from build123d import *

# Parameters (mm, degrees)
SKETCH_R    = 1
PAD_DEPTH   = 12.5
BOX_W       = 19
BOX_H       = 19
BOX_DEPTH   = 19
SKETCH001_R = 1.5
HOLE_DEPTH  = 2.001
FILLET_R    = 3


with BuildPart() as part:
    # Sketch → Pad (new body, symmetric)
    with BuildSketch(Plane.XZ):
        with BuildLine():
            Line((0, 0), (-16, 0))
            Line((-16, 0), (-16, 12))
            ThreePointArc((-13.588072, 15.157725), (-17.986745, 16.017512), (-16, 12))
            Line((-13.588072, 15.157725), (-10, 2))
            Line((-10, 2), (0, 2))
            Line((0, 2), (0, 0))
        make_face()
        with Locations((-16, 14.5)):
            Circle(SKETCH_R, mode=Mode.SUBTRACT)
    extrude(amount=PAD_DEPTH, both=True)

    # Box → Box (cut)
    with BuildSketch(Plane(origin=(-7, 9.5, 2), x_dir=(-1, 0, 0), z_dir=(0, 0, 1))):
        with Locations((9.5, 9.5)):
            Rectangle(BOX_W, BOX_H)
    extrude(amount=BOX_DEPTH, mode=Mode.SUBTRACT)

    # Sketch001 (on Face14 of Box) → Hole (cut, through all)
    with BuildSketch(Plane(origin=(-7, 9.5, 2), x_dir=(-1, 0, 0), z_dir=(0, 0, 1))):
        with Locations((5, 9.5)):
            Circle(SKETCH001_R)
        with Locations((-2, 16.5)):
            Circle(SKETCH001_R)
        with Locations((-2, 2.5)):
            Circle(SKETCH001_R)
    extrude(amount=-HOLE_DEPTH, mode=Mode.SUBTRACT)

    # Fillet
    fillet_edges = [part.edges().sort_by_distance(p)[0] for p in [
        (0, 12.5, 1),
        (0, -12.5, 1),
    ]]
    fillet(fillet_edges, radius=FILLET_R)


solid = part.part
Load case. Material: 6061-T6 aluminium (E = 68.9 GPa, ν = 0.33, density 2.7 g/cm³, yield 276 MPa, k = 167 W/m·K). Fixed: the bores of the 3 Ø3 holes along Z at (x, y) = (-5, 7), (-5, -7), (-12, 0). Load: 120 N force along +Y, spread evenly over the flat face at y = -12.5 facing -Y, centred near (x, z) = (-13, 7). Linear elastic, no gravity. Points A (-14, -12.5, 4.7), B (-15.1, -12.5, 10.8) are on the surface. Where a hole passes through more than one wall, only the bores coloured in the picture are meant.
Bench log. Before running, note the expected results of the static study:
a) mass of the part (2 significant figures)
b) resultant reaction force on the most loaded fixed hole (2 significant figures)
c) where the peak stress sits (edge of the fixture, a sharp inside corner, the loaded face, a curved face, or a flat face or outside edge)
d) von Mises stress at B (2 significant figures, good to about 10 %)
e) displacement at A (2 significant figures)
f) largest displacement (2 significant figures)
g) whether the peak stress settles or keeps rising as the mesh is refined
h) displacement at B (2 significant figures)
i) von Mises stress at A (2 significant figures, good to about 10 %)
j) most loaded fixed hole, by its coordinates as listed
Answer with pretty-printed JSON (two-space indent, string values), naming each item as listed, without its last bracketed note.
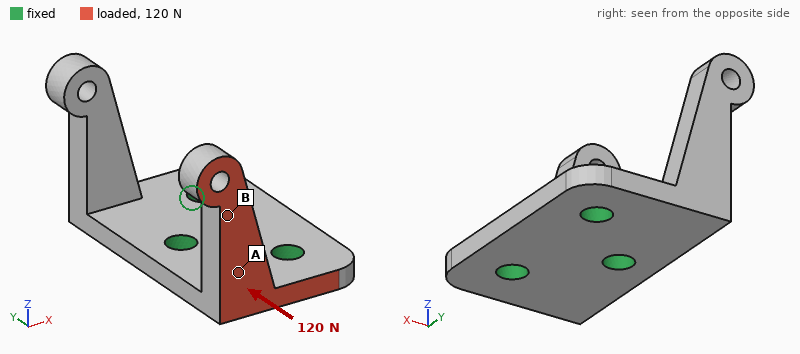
{
  "mass of the part": "3.1 g",
  "resultant reaction force on the most loaded fixed hole": "100 N",
  "where the peak stress sits": "edge of the fixture",
  "von Mises stress at B": "19 MPa",
  "displacement at A": "0.050 mm",
  "largest displacement": "0.17 mm",
  "whether the peak stress settles or keeps rising as the mesh is refined": "keeps rising",
  "displacement at B": "0.10 mm",
  "von Mises stress at A": "48 MPa",
  "most loaded fixed hole, by its coordinates as listed": "(-12, 0)"
}
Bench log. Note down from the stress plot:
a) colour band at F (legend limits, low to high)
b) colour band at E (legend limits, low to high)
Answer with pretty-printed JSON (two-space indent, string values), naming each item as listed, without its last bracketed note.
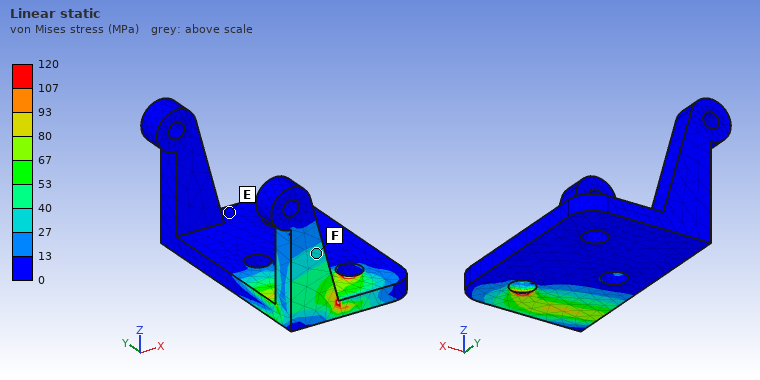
{
  "colour band at F": "27 to 40 MPa",
  "colour band at E": "0 to 13 MPa"
}
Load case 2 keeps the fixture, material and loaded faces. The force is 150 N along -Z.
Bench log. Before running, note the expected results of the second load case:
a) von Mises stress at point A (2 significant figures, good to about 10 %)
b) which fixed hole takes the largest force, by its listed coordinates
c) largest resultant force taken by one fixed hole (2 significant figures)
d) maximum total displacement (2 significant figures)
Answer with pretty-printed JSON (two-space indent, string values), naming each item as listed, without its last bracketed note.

{
  "von Mises stress at point A": "21 MPa",
  "which fixed hole takes the largest force, by its listed coordinates": "(-5, -7)",
  "largest resultant force taken by one fixed hole": "120 N",
  "maximum total displacement": "0.19 mm"
}
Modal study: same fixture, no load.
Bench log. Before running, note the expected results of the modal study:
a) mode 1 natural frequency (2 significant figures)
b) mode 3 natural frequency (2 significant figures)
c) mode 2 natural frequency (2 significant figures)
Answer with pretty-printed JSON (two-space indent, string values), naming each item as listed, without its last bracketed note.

{
  "mode 1 natural frequency": "5400 Hz",
  "mode 3 natural frequency": "8100 Hz",
  "mode 2 natural frequency": "5500 Hz"
}
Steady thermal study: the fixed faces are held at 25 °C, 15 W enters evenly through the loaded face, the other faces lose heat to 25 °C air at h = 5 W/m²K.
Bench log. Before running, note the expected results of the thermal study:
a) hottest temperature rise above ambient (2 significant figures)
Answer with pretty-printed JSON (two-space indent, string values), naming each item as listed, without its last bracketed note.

{
  "hottest temperature rise above ambient": "64 K"
}
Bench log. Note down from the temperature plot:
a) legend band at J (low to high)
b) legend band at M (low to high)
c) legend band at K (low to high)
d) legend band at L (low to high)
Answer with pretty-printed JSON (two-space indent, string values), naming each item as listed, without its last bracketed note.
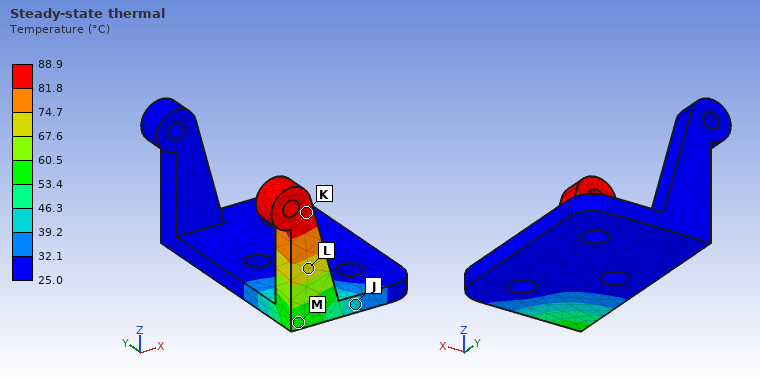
{
  "legend band at J": "39.2 to 46.3 °C",
  "legend band at M": "53.4 to 60.5 °C",
  "legend band at K": "81.8 to 88.9 °C",
  "legend band at L": "67.6 to 74.7 °C"
}
